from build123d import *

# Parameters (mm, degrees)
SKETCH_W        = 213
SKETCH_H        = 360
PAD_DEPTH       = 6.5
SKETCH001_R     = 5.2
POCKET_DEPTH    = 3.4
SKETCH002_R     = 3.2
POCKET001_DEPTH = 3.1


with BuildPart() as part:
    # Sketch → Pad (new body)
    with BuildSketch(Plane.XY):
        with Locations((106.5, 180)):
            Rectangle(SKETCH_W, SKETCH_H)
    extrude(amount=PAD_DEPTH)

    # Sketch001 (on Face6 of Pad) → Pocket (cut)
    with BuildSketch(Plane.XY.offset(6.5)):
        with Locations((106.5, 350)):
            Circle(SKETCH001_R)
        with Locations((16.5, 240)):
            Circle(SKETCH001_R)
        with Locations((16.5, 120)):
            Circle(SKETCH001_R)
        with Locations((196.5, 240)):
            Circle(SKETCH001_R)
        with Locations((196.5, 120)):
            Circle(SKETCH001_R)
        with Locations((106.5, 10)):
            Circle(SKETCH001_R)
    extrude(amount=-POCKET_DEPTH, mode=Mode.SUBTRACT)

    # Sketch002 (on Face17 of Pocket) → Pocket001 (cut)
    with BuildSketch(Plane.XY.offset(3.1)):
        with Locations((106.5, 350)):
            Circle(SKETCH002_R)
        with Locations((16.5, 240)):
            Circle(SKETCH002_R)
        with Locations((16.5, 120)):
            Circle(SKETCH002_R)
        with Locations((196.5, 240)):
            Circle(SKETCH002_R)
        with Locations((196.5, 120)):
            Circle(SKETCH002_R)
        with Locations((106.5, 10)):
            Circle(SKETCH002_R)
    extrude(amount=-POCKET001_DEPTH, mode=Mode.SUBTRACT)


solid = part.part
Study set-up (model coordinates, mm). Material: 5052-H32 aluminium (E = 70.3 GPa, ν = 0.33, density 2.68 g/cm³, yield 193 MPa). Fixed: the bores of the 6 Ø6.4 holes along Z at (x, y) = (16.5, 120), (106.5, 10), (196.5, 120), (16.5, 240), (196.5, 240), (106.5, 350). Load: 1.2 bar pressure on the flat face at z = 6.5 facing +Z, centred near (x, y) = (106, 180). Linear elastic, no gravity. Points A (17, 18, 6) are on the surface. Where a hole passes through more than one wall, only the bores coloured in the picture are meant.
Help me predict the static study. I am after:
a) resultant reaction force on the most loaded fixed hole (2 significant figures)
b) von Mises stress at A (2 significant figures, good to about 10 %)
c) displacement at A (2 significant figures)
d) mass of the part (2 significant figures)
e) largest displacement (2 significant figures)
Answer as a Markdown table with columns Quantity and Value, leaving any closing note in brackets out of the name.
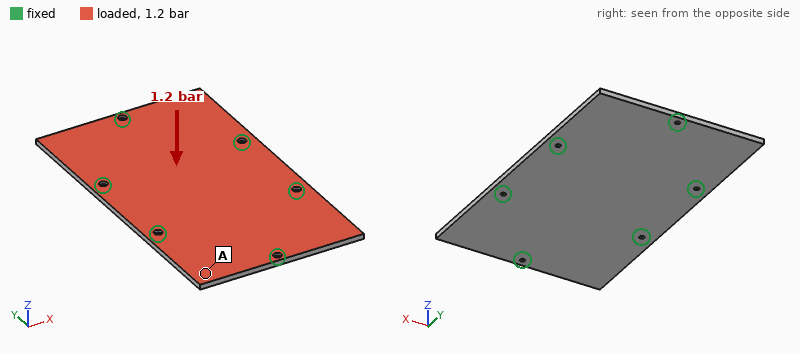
| Quantity | Value |
|---|---|
| resultant reaction force on the most loaded fixed hole | 2.4 kN |
| von Mises stress at A | 15 MPa |
| displacement at A | 0.30 mm |
| mass of the part | 1.3 kg |
| largest displacement | 0.39 mm |
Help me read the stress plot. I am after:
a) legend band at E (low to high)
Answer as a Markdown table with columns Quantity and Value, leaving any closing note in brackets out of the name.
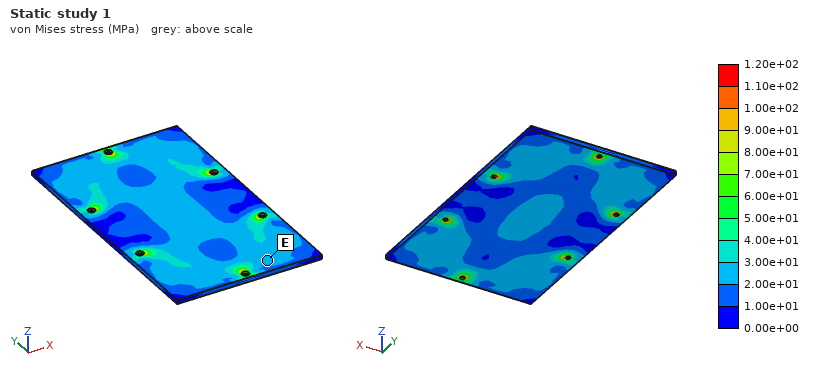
| Quantity | Value |
|---|---|
| legend band at E | 2.00e+01 to 3.00e+01 MPa |
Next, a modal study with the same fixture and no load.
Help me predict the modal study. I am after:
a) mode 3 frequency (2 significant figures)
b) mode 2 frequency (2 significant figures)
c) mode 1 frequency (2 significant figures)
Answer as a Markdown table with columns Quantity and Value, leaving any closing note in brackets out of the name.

| Quantity | Value |
|---|---|
| mode 3 frequency | 730 Hz |
| mode 2 frequency | 690 Hz |
| mode 1 frequency | 680 Hz |
